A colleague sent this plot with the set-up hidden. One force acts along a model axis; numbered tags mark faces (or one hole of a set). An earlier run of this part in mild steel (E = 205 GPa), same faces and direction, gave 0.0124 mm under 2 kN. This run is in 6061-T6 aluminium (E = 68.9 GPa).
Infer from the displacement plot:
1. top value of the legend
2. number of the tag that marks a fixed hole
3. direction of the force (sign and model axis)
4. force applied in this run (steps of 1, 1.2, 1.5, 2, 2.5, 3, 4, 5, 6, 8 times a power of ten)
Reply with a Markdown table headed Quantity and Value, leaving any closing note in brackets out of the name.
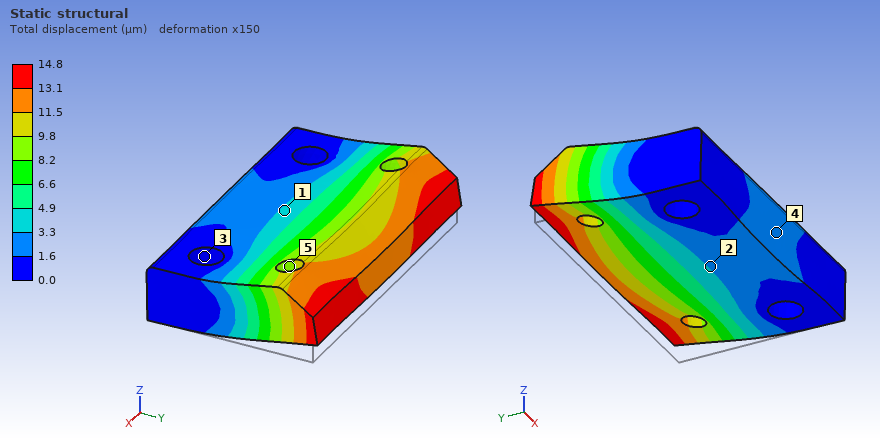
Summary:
| Quantity | Value |
|---|---|
| top value of the legend | 14.8 µm |
| number of the tag that marks a fixed hole | 3 |
| direction of the force | +Z |
| force applied in this run | 800 N |
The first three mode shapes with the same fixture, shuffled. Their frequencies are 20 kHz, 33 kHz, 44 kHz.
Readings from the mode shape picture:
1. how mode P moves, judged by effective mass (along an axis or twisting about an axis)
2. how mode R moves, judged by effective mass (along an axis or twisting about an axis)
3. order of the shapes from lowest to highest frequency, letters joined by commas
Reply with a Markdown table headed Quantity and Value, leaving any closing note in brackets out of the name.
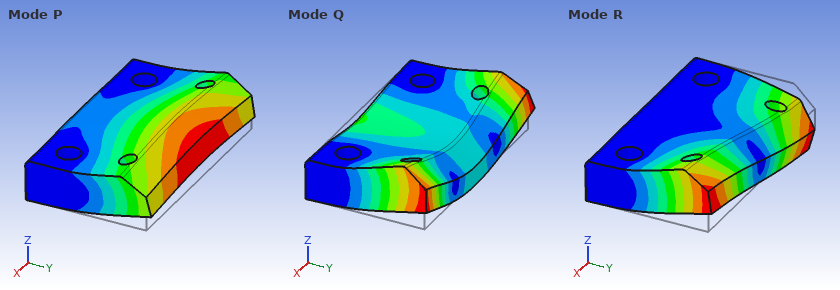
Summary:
| Quantity | Value |
|---|---|
| how mode P moves, judged by effective mass | along Z |
| how mode R moves, judged by effective mass | twisting about Y |
| order of the shapes from lowest to highest frequency, letters joined by commas | P, R, Q |
